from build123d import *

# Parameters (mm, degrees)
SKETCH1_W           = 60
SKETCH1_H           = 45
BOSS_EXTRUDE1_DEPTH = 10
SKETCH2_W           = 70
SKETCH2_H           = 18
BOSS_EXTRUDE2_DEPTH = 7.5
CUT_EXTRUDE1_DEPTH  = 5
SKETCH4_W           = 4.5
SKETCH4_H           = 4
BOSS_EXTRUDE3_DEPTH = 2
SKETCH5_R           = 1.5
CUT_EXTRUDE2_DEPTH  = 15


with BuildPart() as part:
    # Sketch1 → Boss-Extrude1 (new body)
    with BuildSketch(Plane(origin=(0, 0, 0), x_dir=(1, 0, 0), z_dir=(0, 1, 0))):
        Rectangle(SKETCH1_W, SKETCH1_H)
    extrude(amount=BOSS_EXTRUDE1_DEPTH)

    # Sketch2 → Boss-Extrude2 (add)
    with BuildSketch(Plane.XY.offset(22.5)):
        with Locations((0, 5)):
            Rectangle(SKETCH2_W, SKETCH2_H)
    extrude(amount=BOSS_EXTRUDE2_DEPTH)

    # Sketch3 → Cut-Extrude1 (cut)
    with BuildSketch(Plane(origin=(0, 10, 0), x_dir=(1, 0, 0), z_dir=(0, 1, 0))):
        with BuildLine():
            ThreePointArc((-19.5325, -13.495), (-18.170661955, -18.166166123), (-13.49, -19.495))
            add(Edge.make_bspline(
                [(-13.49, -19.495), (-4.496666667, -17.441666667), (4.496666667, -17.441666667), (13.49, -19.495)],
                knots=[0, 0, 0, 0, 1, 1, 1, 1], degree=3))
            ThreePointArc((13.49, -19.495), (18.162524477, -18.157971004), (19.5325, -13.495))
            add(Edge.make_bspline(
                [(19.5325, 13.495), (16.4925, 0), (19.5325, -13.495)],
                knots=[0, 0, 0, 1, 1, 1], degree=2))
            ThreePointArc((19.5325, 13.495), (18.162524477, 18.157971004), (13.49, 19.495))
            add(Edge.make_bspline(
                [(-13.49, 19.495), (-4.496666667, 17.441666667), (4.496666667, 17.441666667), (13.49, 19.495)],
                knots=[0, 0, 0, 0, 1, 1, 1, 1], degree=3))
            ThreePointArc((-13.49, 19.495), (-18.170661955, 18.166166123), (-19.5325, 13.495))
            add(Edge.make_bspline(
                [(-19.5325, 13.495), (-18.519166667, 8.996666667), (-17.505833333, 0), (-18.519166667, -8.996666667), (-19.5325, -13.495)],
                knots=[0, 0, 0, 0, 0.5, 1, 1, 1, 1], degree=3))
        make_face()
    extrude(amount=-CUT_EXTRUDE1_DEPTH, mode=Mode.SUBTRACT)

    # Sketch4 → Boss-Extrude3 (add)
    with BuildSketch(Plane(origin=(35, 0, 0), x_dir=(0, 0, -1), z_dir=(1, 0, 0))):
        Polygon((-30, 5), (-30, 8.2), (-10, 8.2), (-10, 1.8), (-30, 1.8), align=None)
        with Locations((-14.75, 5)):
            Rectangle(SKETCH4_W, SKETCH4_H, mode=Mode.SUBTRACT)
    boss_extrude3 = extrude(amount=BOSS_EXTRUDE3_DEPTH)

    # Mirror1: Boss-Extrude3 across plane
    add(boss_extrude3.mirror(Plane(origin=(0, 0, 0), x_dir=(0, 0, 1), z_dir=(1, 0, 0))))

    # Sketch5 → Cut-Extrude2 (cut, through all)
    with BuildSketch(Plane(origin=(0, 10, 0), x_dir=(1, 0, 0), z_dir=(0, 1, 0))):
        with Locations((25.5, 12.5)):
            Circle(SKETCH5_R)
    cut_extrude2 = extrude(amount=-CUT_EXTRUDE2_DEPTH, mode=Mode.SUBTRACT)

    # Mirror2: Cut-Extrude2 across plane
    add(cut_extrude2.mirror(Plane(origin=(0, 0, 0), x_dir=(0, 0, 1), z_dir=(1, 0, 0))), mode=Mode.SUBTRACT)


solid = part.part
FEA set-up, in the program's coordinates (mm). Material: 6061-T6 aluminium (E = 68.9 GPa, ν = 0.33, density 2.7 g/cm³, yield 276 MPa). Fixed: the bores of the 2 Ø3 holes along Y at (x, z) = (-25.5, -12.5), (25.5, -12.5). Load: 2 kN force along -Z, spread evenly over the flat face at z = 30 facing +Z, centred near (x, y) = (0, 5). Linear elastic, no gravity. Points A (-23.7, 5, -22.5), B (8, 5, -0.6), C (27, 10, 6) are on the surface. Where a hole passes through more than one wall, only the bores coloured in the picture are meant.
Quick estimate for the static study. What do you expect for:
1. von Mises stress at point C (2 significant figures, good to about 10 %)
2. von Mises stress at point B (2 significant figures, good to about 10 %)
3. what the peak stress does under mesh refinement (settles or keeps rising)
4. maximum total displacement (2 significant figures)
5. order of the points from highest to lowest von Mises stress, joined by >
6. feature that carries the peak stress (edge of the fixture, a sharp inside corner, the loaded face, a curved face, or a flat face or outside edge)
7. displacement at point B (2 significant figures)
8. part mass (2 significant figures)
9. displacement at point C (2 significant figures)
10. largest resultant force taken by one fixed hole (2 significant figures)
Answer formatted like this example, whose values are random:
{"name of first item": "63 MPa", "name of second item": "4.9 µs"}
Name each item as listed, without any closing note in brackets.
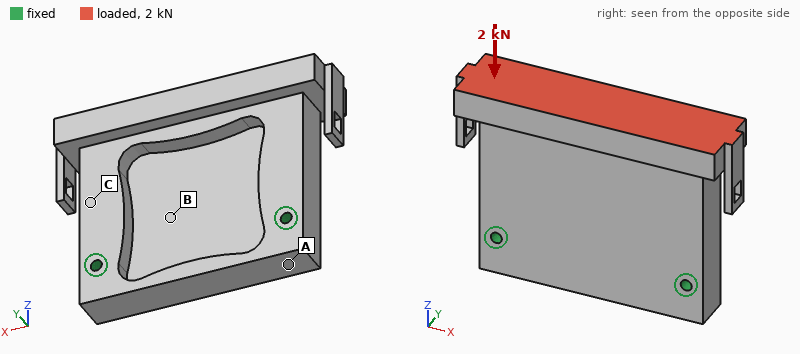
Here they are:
{"von Mises stress at point C": "9.5 MPa", "von Mises stress at point B": "3.7 MPa", "what the peak stress does under mesh refinement": "keeps rising", "maximum total displacement": "10.0 µm", "order of the points from highest to lowest von Mises stress, joined by >": "C > B > A", "feature that carries the peak stress": "edge of the fixture", "displacement at point B": "2.4 µm", "part mass": "80 g", "displacement at point C": "2.8 µm", "largest resultant force taken by one fixed hole": "1.0 kN"}
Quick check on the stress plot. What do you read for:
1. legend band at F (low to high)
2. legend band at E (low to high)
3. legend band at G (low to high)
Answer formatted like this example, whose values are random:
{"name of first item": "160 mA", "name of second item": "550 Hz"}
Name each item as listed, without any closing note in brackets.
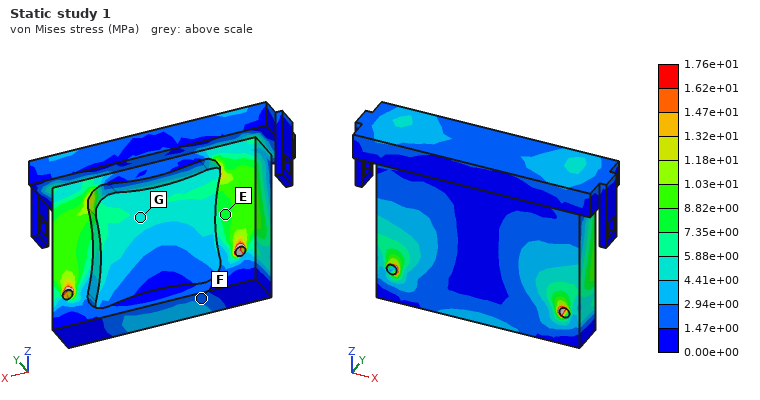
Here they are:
{"legend band at F": "1.47e+00 to 2.94e+00 MPa", "legend band at E": "7.35e+00 to 8.82e+00 MPa", "legend band at G": "4.41e+00 to 5.88e+00 MPa"}
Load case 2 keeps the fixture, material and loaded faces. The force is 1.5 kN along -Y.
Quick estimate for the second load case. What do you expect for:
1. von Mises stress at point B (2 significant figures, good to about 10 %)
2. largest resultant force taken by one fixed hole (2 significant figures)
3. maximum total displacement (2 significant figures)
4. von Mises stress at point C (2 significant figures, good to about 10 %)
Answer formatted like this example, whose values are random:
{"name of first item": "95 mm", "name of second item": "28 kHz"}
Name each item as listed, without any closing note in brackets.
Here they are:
{"von Mises stress at point B": "33 MPa", "largest resultant force taken by one fixed hole": "750 N", "maximum total displacement": "0.27 mm", "von Mises stress at point C": "74 MPa"}
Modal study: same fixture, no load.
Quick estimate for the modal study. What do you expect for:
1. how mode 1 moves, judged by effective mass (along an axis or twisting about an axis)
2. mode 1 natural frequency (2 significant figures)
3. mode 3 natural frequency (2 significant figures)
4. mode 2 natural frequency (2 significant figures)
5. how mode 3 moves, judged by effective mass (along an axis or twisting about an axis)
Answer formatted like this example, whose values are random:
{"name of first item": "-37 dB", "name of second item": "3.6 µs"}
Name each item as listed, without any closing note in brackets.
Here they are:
{"how mode 1 moves, judged by effective mass": "along Y", "mode 1 natural frequency": "2300 Hz", "mode 3 natural frequency": "9000 Hz", "mode 2 natural frequency": "4300 Hz", "how mode 3 moves, judged by effective mass": "along X"}
